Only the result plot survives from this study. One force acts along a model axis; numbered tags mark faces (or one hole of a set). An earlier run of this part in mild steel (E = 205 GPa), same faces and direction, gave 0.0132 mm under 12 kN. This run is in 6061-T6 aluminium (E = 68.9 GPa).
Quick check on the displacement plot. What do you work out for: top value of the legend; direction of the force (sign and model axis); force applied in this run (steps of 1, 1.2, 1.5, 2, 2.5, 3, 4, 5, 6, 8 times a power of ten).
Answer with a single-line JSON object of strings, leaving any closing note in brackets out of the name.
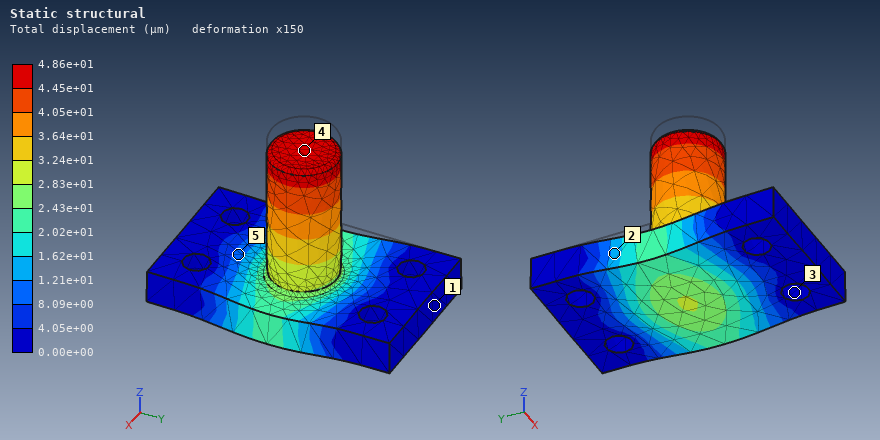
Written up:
{"top value of the legend": "4.86e+01 µm", "direction of the force": "-Z", "force applied in this run": "15 kN"}
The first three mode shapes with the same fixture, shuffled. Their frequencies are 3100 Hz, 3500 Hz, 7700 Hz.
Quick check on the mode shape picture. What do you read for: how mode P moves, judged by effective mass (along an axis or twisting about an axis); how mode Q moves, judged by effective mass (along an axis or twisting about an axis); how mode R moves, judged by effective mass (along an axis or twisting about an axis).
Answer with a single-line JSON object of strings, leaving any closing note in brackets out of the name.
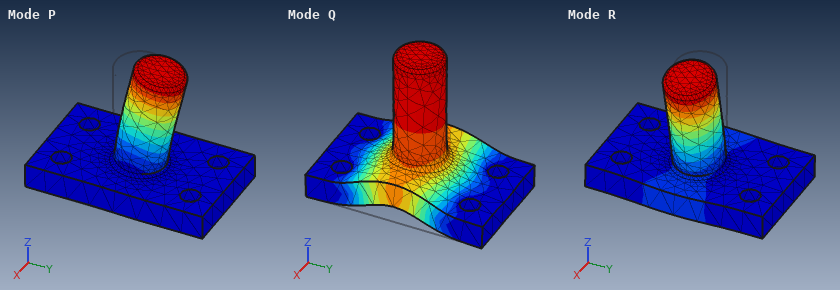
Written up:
{"how mode P moves, judged by effective mass": "along Y", "how mode Q moves, judged by effective mass": "along Z", "how mode R moves, judged by effective mass": "along X"}
